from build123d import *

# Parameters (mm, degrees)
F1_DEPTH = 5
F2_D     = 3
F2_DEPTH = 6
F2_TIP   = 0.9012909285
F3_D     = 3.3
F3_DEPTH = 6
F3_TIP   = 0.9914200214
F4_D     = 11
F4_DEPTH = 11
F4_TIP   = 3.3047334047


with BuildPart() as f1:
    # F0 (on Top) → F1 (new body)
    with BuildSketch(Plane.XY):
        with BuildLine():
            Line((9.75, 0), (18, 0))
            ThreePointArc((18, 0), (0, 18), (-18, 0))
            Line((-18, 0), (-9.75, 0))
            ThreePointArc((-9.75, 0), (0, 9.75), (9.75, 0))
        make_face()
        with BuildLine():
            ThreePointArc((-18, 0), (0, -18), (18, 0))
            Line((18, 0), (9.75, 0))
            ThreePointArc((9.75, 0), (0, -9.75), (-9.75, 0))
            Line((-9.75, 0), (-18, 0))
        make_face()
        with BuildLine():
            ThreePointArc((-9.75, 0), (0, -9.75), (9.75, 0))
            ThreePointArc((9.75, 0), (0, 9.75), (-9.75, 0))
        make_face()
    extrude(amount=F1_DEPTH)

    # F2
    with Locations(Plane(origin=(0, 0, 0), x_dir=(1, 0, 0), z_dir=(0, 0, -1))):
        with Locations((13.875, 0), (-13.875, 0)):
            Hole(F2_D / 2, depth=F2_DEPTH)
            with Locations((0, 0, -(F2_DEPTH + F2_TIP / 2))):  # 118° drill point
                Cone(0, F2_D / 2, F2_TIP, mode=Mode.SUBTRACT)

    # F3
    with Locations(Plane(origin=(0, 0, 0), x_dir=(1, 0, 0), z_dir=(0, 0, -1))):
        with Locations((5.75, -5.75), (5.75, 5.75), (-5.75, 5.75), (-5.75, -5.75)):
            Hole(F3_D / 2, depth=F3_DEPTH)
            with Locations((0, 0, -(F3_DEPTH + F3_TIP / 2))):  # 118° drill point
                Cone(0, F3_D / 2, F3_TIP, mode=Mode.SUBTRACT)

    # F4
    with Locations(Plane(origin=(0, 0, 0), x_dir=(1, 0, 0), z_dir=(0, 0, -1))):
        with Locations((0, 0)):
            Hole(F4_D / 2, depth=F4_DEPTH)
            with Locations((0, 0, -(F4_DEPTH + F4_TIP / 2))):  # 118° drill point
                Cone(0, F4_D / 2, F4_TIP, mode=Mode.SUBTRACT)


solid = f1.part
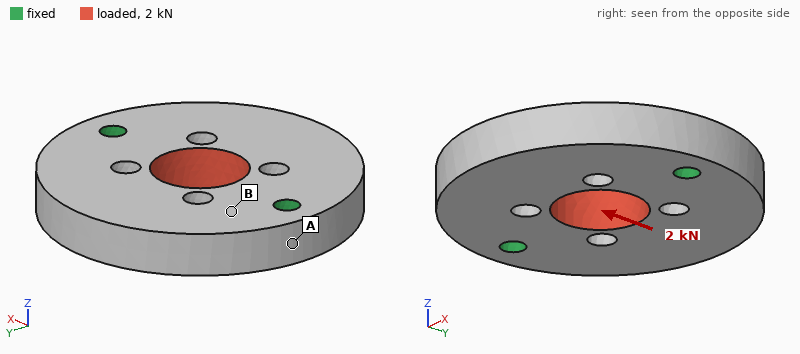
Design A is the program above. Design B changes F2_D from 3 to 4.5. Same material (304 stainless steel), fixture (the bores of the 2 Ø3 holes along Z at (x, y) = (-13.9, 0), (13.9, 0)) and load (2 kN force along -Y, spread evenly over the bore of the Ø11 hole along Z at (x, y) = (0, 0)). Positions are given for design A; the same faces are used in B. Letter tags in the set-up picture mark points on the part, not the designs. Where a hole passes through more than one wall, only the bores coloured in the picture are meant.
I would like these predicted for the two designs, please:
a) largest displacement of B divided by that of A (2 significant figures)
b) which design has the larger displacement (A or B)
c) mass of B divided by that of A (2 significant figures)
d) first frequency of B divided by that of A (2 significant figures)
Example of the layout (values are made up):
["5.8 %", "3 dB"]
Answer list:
["0.91", "A", "0.98", "1.1"]
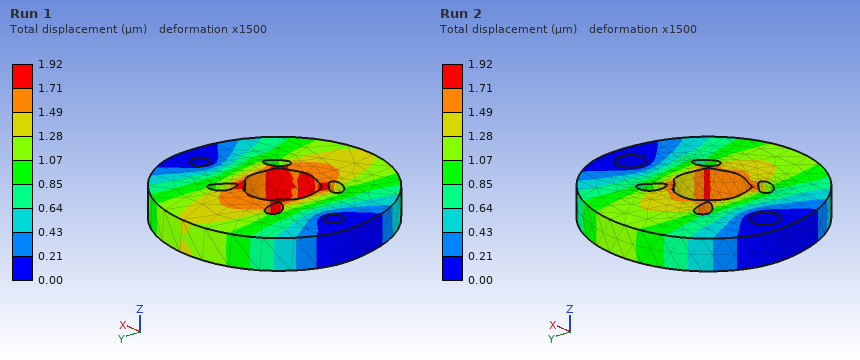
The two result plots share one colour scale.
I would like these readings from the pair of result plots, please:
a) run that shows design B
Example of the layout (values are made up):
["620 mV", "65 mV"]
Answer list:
["Run 2"]
